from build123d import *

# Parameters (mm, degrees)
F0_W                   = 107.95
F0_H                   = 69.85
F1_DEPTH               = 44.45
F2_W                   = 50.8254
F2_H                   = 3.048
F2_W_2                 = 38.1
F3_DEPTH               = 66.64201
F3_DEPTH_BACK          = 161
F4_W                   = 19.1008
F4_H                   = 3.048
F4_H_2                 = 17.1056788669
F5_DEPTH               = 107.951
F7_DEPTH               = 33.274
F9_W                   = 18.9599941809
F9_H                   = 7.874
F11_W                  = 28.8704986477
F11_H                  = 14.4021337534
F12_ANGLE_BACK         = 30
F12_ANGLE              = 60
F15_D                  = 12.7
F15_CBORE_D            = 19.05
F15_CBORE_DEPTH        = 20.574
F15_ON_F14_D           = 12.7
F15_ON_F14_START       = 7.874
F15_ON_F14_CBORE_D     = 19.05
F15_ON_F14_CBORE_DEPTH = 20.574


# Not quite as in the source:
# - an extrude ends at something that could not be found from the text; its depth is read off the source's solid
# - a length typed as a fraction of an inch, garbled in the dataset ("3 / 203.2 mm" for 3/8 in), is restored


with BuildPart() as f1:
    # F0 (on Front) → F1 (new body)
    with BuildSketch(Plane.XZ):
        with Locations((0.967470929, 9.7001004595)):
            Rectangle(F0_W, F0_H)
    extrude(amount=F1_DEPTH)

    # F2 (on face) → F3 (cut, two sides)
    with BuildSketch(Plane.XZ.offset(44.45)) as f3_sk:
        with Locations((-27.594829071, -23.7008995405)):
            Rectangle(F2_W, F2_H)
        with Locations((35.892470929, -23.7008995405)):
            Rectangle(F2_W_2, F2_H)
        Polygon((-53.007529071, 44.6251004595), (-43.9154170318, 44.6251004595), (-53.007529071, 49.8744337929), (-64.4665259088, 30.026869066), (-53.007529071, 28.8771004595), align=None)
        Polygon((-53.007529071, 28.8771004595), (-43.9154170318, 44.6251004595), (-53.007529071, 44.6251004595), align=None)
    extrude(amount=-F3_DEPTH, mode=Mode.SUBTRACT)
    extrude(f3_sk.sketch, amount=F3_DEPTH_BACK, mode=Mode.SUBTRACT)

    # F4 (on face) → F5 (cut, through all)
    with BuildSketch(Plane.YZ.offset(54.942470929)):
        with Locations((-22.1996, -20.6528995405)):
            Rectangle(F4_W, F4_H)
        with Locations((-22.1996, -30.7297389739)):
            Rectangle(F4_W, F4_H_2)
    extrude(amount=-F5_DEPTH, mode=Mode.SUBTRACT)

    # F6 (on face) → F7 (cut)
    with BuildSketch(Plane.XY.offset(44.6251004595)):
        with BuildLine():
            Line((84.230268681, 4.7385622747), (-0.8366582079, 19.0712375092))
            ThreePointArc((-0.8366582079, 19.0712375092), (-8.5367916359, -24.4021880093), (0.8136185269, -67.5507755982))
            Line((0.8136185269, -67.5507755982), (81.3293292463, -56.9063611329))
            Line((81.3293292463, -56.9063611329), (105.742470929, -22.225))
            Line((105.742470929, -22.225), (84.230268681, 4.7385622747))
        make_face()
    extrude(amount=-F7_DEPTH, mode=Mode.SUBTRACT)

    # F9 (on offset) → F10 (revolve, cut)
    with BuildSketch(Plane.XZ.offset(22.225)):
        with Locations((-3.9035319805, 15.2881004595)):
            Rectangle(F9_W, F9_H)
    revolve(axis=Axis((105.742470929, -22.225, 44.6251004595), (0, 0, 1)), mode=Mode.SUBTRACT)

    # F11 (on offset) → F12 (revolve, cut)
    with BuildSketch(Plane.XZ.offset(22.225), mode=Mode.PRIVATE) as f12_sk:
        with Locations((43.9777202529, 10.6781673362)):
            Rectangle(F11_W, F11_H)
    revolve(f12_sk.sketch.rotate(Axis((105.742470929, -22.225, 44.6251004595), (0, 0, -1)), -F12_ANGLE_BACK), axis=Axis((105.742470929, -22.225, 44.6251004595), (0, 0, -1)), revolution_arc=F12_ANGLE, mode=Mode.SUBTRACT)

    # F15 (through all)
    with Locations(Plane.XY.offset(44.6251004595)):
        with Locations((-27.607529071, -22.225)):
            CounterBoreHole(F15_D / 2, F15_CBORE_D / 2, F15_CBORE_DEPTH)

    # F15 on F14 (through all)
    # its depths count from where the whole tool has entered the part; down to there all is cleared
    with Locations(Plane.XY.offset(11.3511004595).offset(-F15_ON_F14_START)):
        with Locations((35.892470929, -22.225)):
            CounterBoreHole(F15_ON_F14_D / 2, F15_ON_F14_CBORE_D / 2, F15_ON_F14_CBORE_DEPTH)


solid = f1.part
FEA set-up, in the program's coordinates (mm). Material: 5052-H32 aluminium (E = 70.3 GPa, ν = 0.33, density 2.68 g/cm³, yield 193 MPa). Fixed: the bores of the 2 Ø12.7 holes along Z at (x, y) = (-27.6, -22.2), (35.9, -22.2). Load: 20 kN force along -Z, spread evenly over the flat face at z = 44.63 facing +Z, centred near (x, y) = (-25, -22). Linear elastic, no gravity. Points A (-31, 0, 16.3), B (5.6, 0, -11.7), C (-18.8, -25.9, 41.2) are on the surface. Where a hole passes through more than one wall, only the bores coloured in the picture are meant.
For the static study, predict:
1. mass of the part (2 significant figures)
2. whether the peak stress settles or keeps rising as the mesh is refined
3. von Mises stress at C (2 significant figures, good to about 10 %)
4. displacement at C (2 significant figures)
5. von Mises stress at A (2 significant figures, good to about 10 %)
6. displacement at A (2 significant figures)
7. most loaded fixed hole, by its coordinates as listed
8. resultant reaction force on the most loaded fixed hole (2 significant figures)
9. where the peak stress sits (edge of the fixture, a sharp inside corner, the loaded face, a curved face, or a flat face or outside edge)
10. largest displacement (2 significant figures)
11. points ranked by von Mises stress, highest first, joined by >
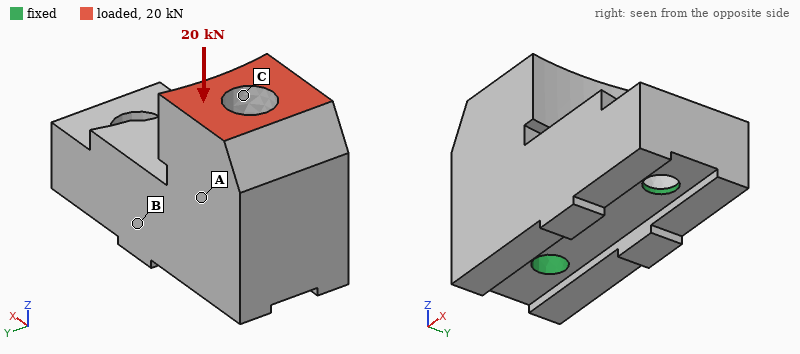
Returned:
510 g
keeps rising
18 MPa
11 µm
9.3 MPa
4.2 µm
(-27.6, -22.2)
20 kN
edge of the fixture
16 µm
C > A > B
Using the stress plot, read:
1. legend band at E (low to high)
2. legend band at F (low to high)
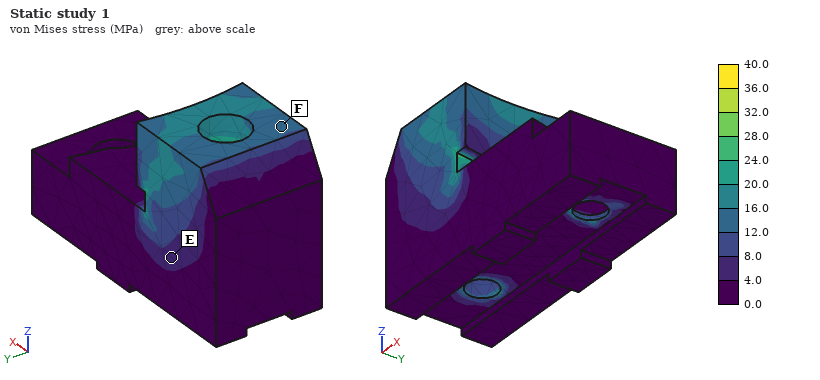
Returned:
4.0 to 8.0 MPa
12.0 to 16.0 MPa
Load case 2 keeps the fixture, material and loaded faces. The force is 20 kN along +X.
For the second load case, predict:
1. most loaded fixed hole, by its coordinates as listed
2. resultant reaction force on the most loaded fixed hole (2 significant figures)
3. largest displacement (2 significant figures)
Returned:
(-27.6, -22.2)
20 kN
69 µm
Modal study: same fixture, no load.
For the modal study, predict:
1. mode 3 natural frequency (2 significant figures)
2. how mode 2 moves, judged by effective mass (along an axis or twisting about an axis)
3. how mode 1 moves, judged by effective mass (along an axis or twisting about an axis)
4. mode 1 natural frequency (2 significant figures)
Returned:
13 kHz
along Z
along Y
7800 Hz
